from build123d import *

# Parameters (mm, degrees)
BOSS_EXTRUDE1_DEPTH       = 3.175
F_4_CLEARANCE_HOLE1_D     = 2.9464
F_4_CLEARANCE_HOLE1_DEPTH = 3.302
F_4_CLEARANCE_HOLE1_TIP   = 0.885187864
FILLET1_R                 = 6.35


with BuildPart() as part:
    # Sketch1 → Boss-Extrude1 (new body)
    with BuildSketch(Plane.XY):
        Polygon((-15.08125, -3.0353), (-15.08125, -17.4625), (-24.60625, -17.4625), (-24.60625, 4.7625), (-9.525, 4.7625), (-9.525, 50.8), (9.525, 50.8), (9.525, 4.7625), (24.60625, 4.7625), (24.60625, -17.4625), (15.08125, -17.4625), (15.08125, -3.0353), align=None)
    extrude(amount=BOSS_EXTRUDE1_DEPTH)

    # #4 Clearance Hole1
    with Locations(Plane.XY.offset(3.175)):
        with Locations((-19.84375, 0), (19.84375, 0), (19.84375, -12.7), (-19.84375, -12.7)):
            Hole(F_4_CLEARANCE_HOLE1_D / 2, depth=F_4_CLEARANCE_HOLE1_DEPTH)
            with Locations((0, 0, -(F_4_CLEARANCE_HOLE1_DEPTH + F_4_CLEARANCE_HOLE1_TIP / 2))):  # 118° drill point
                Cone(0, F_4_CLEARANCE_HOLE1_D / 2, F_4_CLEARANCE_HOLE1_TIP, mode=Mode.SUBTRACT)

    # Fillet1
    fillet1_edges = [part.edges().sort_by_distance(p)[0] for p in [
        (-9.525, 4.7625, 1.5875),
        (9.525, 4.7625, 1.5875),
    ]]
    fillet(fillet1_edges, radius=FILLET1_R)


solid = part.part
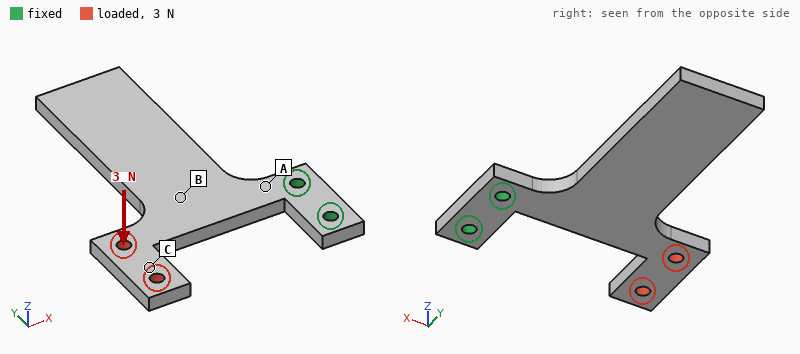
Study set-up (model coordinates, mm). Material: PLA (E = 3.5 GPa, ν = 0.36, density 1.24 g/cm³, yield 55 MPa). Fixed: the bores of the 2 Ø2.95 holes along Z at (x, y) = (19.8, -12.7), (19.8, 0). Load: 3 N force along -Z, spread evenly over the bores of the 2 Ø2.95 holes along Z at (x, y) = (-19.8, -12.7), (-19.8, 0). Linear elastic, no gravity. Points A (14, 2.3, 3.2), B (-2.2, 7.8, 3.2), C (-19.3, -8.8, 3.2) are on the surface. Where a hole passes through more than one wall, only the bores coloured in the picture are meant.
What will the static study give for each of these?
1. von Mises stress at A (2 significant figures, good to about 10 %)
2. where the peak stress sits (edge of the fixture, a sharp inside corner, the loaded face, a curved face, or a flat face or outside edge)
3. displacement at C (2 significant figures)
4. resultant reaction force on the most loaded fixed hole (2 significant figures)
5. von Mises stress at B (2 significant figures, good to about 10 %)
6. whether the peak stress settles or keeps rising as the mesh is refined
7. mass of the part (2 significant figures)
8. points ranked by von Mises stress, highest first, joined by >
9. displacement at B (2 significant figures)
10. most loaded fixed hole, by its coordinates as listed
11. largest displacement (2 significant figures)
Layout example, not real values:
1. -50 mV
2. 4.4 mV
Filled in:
1. 7.0 MPa
2. edge of the fixture
3. 0.68 mm
4. 3.6 N
5. 1.7 MPa
6. keeps rising
7. 6.0 g
8. A > B > C
9. 0.23 mm
10. (19.8, 0)
11. 0.88 mm
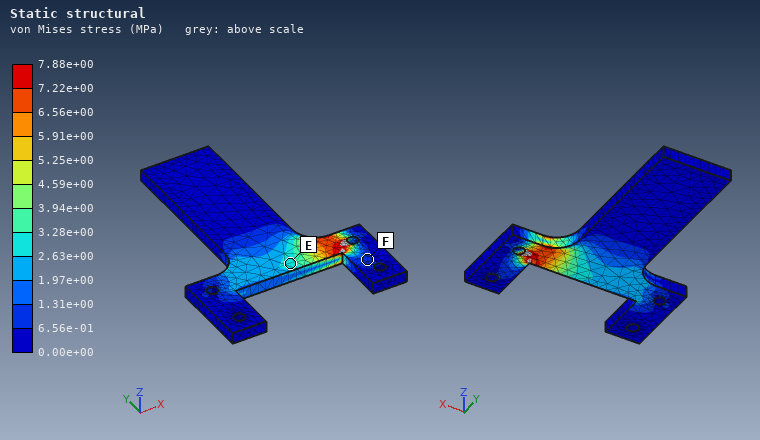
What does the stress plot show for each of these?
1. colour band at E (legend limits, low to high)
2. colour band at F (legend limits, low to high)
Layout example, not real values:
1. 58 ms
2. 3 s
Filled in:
1. 2.63e+00 to 3.28e+00 MPa
2. 6.56e-01 to 1.31e+00 MPa
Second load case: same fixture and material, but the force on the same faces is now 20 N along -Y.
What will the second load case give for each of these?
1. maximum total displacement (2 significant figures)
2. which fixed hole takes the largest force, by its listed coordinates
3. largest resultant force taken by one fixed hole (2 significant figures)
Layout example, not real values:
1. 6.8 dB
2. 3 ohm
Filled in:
1. 0.91 mm
2. (19.8, -12.7)
3. 50 N
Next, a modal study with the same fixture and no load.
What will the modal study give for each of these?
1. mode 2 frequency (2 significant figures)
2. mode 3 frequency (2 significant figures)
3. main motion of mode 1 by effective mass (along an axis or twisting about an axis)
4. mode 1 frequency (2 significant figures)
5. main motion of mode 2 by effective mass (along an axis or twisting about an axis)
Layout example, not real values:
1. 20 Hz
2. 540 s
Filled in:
1. 320 Hz
2. 440 Hz
3. along Z
4. 200 Hz
5. along Z
